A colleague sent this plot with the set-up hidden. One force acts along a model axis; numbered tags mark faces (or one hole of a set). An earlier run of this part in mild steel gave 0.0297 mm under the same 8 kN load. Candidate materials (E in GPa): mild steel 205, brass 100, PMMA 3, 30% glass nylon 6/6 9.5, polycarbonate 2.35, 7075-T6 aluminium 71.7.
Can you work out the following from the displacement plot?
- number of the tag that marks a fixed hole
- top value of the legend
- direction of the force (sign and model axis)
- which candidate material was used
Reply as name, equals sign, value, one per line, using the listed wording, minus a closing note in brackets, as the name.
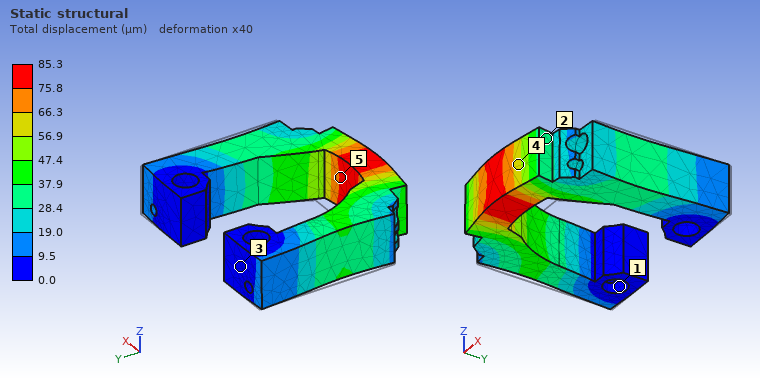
number of the tag that marks a fixed hole = 1
top value of the legend = 85.3 µm
direction of the force = -Y
which candidate material was used = 7075-T6 aluminium
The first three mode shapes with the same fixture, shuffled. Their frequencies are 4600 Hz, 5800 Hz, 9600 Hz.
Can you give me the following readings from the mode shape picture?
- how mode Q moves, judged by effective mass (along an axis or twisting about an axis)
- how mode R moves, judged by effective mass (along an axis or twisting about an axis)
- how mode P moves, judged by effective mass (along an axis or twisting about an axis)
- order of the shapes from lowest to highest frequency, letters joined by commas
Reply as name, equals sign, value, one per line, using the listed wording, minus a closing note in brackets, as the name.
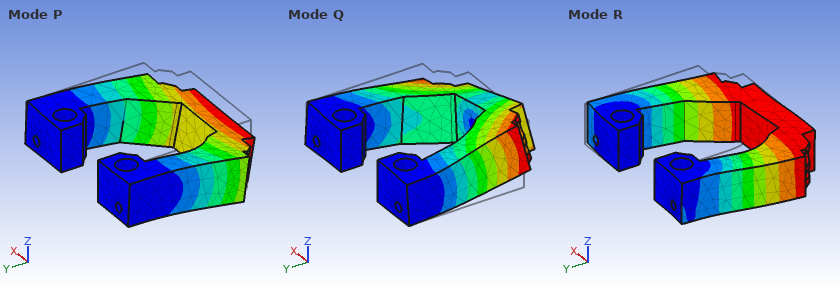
how mode Q moves, judged by effective mass = twisting about Y
how mode R moves, judged by effective mass = along X
how mode P moves, judged by effective mass = along Z
order of the shapes from lowest to highest frequency, letters joined by commas = P, R, Q
